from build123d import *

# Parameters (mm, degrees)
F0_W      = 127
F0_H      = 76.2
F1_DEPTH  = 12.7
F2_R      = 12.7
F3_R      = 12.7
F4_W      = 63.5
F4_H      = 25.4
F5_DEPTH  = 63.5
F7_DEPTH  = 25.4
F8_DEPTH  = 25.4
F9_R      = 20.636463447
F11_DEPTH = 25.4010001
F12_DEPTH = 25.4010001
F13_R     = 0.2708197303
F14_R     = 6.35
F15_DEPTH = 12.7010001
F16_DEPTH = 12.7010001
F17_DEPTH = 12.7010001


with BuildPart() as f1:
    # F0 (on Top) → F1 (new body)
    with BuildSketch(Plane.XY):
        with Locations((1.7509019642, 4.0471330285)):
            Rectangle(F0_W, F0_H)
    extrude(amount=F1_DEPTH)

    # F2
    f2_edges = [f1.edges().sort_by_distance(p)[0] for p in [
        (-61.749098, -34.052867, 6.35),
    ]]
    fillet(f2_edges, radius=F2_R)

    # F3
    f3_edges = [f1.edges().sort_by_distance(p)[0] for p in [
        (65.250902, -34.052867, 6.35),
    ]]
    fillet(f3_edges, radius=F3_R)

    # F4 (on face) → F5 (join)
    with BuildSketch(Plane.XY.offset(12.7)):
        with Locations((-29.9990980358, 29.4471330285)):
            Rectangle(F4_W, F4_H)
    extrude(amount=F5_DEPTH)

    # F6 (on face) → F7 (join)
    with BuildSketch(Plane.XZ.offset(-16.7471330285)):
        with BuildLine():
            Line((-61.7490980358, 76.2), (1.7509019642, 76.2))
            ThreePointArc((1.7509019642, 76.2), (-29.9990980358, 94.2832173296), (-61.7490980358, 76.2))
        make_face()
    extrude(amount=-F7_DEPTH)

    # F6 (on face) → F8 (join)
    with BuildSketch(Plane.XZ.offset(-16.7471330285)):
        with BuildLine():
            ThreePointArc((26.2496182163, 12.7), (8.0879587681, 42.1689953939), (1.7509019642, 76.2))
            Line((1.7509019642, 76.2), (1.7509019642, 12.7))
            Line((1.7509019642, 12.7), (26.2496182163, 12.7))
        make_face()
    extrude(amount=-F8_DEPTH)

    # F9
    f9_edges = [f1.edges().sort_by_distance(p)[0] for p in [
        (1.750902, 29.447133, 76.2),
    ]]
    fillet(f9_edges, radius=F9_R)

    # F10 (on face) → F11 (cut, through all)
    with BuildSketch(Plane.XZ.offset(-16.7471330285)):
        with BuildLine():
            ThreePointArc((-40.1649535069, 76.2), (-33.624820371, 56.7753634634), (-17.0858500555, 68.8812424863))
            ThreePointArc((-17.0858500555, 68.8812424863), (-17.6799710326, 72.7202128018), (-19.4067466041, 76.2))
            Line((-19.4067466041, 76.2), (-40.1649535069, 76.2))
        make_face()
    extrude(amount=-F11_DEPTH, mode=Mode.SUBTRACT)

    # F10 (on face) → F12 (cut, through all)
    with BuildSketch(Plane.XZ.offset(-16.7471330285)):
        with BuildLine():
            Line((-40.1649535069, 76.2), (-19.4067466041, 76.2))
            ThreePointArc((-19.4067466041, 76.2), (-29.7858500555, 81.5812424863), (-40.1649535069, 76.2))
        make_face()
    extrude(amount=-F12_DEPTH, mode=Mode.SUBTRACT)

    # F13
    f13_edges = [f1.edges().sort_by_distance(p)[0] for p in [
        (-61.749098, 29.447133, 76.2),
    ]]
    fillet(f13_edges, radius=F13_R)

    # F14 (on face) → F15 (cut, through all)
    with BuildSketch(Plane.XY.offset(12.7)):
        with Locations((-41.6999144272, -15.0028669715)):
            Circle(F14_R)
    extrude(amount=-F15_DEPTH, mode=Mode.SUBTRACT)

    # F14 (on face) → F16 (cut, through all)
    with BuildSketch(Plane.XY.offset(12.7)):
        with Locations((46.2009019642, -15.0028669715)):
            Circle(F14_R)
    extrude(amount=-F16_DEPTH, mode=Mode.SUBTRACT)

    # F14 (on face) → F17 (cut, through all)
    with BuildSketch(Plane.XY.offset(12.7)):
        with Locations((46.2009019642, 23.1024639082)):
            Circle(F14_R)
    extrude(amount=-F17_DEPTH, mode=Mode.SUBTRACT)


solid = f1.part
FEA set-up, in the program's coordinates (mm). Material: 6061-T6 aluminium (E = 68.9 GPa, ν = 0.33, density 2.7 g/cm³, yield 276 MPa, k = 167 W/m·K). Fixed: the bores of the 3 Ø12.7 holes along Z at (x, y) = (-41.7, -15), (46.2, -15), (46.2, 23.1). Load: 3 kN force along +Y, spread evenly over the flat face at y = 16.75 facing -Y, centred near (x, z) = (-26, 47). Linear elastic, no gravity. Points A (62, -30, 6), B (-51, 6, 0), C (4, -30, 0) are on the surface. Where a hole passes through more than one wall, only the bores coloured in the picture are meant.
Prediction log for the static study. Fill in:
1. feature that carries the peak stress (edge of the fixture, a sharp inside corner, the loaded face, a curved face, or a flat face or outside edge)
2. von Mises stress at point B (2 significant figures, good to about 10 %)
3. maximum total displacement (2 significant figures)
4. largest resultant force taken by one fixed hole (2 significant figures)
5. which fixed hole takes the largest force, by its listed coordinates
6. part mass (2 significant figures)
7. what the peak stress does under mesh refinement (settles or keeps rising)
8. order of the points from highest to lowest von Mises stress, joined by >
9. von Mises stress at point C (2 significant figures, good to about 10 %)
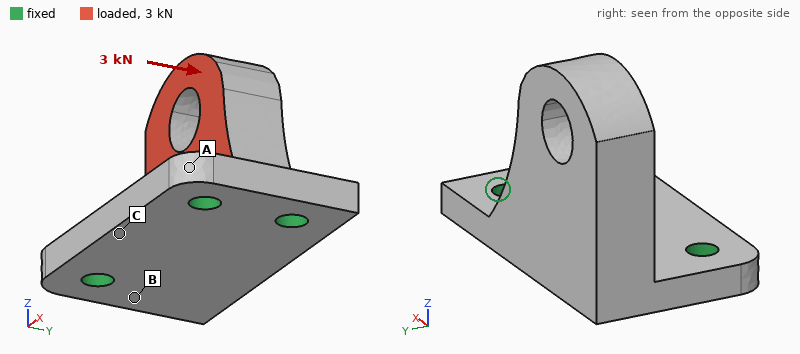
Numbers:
edge of the fixture
24 MPa
0.23 mm
2.1 kN
(-41.7, -15)
650 g
keeps rising
B > C > A
8.6 MPa
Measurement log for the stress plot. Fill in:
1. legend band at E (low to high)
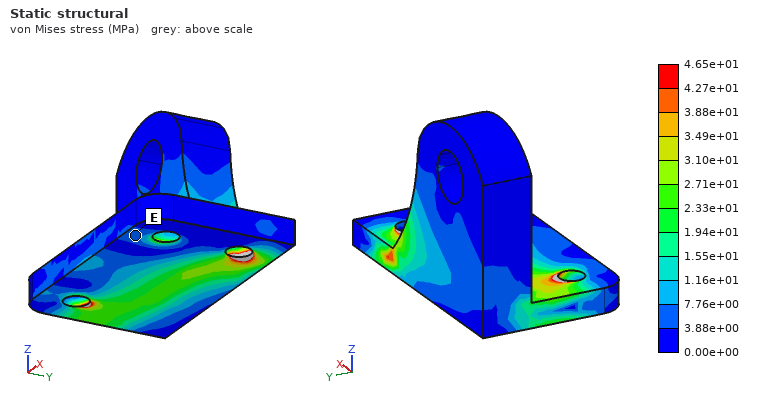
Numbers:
3.88e+00 to 7.76e+00 MPa
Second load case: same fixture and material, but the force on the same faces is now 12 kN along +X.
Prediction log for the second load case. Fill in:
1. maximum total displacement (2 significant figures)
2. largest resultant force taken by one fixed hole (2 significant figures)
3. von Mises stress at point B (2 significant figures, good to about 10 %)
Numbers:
0.35 mm
7.6 kN
36 MPa
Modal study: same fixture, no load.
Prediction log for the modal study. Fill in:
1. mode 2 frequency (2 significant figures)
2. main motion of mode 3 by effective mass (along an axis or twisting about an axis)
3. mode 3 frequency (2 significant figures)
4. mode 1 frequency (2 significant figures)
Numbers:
2600 Hz
along Z
4400 Hz
1100 Hz
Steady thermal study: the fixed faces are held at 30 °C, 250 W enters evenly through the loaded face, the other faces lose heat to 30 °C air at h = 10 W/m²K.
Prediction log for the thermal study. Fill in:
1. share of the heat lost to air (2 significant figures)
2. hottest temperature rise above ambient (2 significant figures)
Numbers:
4.3 %
77 K
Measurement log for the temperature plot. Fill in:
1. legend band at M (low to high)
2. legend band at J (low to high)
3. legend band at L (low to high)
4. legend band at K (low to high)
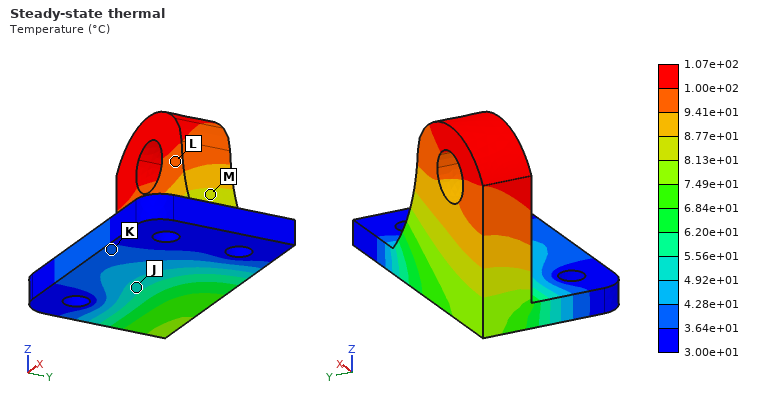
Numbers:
8.13e+01 to 8.77e+01 °C
4.92e+01 to 5.56e+01 °C
9.41e+01 to 1.00e+02 °C
3.64e+01 to 4.28e+01 °C
